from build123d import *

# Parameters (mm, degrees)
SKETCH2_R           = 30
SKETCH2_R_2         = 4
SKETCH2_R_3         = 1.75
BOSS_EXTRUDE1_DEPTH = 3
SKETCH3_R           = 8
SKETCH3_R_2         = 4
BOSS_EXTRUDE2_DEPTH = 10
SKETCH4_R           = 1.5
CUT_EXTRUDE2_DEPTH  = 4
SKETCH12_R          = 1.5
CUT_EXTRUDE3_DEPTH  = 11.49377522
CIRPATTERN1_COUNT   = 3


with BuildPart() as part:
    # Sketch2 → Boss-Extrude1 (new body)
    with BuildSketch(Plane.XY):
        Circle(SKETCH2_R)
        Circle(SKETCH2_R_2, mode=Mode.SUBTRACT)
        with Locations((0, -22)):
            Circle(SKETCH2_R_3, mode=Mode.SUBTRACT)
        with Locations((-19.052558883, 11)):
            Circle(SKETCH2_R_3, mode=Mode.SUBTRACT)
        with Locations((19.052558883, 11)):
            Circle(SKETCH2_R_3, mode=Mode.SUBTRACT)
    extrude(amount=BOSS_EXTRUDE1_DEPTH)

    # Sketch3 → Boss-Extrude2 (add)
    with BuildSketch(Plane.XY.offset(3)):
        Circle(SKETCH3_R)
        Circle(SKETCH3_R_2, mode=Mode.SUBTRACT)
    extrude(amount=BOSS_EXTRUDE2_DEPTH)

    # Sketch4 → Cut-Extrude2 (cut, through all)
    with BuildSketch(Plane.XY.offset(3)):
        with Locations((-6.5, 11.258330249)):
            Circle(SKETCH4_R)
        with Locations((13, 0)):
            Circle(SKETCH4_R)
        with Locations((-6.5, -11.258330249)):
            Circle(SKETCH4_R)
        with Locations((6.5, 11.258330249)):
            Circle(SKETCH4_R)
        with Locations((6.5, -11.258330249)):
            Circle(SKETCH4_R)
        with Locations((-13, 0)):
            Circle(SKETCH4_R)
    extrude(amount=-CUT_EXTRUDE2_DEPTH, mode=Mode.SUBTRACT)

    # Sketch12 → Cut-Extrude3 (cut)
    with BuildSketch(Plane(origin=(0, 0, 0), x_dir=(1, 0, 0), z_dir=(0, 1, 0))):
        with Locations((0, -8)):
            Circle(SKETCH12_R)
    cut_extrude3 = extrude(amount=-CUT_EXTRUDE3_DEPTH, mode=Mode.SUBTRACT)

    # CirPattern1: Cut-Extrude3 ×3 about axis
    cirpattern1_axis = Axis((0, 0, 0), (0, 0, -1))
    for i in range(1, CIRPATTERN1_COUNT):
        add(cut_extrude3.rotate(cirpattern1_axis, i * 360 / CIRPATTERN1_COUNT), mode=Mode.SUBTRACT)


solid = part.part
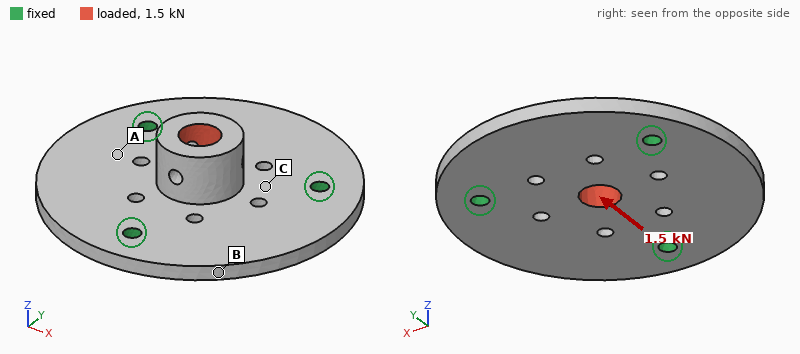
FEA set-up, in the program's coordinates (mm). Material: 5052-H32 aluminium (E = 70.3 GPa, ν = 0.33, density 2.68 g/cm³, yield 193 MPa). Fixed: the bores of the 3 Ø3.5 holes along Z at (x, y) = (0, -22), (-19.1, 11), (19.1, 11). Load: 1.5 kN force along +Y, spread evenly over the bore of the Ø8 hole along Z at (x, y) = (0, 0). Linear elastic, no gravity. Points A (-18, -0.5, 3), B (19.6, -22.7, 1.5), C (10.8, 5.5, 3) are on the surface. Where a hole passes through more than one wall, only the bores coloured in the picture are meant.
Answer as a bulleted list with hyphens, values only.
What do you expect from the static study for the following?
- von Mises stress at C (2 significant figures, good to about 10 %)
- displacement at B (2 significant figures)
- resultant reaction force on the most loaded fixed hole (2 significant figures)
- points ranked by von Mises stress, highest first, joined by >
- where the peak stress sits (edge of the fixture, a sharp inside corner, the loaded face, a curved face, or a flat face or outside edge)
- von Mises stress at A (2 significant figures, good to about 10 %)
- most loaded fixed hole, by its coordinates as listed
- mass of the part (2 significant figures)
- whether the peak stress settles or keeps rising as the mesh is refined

- 29 MPa
- 6.1 µm
- 620 N
- C > A > B
- edge of the fixture
- 12 MPa
- (0, -22)
- 26 g
- keeps rising
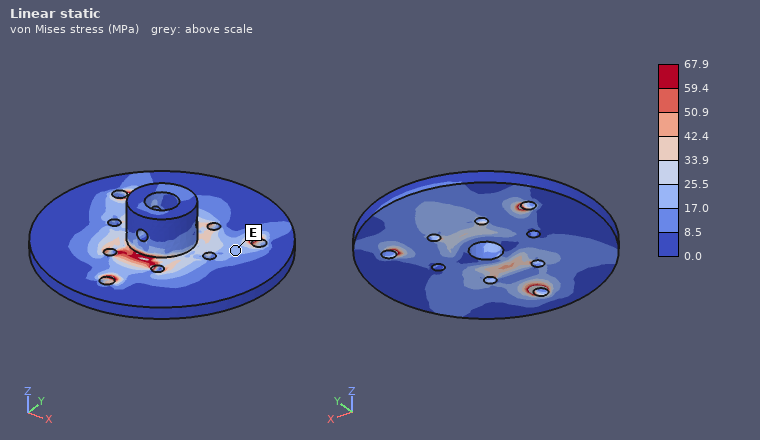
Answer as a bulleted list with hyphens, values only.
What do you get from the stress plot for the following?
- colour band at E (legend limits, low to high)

- 17.0 to 25.5 MPa
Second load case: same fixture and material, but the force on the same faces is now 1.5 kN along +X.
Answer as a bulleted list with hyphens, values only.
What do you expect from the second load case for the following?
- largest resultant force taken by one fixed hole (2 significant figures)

- 580 N
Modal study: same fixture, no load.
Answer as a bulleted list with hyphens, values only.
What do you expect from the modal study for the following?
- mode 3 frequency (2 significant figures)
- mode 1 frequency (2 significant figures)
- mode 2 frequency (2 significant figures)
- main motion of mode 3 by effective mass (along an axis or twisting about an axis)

- 6800 Hz
- 6200 Hz
- 6300 Hz
- along Z
